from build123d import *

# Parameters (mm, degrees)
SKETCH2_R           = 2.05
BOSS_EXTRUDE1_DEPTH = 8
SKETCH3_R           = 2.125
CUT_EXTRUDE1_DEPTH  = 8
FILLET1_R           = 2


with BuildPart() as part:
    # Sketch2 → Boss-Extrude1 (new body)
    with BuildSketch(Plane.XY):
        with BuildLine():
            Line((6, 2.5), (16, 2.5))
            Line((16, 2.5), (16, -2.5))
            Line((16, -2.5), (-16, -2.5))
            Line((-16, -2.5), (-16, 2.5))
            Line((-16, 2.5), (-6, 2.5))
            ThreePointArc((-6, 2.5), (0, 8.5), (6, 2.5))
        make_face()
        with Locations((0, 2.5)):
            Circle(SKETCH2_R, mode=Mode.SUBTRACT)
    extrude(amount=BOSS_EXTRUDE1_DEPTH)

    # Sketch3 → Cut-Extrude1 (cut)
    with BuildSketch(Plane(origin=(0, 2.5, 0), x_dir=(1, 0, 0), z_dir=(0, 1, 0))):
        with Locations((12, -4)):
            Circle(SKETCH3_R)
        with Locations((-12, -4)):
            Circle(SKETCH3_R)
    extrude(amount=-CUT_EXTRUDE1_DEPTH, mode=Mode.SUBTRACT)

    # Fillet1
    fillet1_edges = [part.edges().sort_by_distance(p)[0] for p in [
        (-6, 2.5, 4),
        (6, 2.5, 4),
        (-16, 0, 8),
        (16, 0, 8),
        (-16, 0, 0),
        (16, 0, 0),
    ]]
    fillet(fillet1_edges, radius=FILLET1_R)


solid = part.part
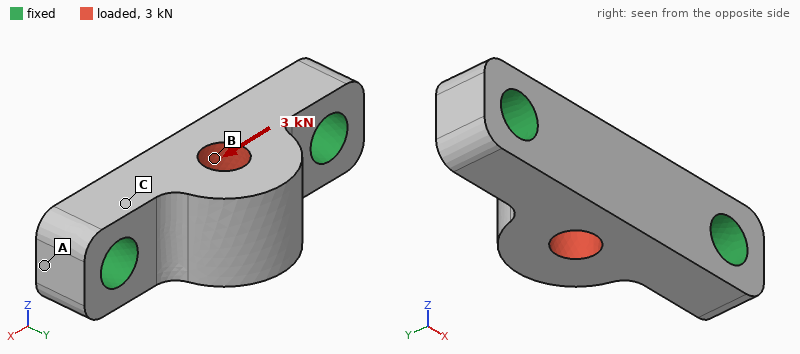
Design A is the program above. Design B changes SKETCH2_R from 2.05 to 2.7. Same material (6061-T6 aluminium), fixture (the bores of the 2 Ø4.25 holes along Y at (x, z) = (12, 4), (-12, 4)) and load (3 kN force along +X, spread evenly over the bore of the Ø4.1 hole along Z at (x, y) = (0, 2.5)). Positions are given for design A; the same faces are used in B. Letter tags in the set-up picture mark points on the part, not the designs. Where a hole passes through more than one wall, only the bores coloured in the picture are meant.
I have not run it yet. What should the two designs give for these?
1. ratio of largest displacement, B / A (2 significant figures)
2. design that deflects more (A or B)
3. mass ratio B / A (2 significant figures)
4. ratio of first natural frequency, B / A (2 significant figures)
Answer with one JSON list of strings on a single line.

["1.2", "B", "0.95", "1.0"]
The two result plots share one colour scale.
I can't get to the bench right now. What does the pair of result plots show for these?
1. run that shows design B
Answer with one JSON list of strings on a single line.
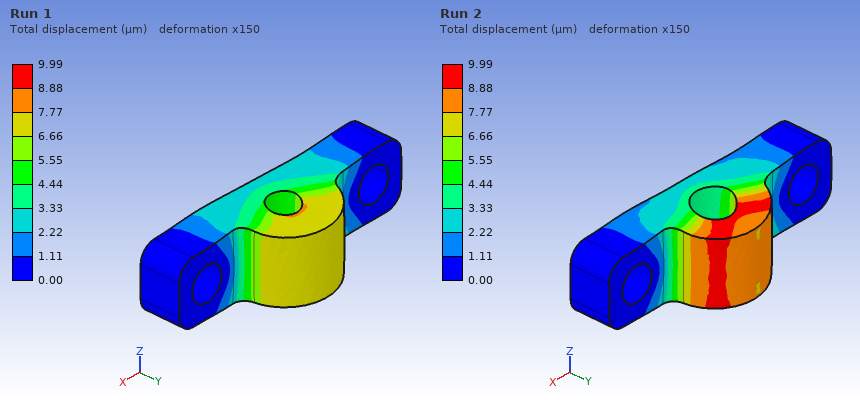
["Run 2"]
